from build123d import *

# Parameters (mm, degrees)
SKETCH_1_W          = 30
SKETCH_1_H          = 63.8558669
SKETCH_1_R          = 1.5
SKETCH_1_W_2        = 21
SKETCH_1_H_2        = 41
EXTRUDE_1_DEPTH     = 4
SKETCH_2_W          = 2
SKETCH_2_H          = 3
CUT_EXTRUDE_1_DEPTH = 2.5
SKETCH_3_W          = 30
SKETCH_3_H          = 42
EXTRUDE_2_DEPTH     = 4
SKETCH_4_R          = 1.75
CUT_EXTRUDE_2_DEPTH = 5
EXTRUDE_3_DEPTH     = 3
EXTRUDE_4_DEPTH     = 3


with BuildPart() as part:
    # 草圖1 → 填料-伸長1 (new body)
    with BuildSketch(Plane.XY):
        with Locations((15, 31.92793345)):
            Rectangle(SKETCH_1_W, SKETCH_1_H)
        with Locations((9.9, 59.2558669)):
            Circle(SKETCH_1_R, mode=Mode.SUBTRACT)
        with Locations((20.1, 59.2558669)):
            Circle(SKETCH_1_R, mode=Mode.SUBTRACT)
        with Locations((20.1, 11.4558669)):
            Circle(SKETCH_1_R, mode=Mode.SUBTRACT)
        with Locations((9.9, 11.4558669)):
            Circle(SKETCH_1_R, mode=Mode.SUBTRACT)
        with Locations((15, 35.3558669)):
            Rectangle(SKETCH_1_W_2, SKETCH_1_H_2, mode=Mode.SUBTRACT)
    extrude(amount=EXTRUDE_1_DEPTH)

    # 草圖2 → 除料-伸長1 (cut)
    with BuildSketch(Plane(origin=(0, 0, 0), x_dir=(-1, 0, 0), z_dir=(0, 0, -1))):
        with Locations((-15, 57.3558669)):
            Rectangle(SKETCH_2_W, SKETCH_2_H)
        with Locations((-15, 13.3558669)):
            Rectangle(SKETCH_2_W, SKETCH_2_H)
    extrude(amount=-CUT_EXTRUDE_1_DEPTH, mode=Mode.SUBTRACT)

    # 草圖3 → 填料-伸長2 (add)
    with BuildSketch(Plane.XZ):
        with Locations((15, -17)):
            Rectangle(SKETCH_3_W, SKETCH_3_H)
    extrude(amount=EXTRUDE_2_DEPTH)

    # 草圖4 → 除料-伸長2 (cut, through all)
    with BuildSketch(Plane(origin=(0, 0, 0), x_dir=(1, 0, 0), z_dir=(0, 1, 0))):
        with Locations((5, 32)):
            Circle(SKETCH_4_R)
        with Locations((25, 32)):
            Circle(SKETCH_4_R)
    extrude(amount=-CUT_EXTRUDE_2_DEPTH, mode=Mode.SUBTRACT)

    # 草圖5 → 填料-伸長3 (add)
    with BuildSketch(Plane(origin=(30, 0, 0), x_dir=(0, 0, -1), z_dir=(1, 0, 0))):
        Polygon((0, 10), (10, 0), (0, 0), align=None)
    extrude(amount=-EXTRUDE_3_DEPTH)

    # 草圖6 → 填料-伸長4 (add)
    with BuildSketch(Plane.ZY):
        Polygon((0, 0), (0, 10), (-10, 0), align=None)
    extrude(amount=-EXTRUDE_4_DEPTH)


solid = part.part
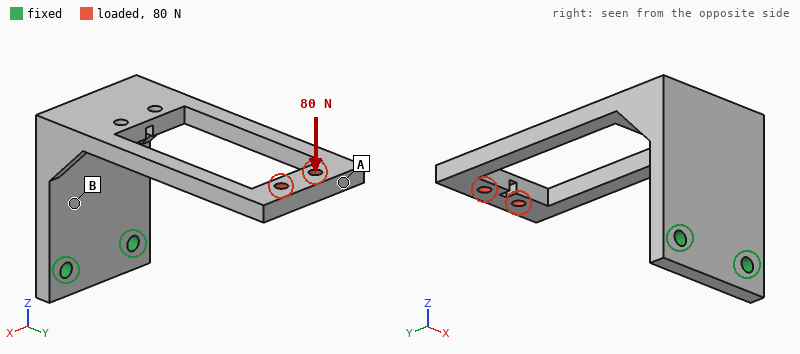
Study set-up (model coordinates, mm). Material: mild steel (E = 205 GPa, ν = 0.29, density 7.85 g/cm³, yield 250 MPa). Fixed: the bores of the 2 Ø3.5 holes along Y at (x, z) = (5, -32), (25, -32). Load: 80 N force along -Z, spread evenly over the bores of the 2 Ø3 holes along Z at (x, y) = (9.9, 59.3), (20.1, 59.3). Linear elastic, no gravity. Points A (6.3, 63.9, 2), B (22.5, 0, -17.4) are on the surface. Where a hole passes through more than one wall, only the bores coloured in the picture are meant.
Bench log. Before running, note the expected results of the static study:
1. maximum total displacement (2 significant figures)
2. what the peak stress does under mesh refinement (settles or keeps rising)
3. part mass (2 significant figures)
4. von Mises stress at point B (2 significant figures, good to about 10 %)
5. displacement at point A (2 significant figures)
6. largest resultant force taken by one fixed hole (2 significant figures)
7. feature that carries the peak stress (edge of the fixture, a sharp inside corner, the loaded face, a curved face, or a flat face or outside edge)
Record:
0.68 mm
keeps rising
73 g
60 MPa
0.67 mm
40 N
a sharp inside corner
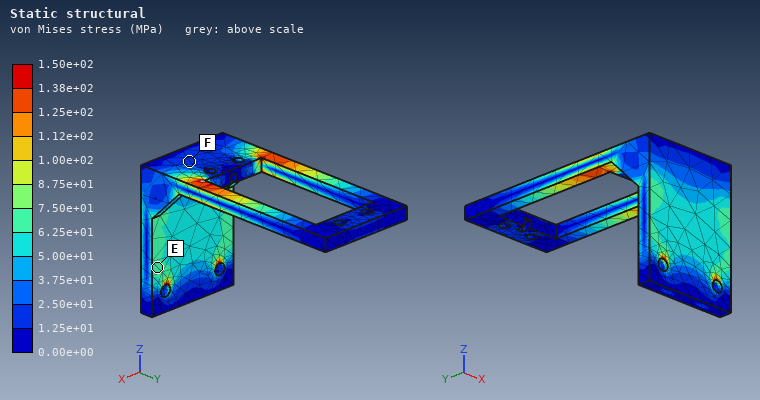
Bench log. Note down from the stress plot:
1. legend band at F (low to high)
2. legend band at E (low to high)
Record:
1.25e+01 to 2.50e+01 MPa
6.25e+01 to 7.50e+01 MPa
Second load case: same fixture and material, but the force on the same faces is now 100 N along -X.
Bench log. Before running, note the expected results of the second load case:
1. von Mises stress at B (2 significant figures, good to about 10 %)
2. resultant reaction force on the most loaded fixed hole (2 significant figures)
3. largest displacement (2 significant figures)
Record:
54 MPa
320 N
0.24 mm
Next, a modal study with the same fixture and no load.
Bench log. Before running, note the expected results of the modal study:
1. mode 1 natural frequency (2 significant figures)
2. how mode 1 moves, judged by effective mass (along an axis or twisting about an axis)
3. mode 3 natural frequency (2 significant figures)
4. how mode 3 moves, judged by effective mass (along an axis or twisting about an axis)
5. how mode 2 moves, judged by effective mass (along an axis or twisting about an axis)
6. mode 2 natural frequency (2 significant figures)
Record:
540 Hz
along Z
1500 Hz
along Y
along X
950 Hz
